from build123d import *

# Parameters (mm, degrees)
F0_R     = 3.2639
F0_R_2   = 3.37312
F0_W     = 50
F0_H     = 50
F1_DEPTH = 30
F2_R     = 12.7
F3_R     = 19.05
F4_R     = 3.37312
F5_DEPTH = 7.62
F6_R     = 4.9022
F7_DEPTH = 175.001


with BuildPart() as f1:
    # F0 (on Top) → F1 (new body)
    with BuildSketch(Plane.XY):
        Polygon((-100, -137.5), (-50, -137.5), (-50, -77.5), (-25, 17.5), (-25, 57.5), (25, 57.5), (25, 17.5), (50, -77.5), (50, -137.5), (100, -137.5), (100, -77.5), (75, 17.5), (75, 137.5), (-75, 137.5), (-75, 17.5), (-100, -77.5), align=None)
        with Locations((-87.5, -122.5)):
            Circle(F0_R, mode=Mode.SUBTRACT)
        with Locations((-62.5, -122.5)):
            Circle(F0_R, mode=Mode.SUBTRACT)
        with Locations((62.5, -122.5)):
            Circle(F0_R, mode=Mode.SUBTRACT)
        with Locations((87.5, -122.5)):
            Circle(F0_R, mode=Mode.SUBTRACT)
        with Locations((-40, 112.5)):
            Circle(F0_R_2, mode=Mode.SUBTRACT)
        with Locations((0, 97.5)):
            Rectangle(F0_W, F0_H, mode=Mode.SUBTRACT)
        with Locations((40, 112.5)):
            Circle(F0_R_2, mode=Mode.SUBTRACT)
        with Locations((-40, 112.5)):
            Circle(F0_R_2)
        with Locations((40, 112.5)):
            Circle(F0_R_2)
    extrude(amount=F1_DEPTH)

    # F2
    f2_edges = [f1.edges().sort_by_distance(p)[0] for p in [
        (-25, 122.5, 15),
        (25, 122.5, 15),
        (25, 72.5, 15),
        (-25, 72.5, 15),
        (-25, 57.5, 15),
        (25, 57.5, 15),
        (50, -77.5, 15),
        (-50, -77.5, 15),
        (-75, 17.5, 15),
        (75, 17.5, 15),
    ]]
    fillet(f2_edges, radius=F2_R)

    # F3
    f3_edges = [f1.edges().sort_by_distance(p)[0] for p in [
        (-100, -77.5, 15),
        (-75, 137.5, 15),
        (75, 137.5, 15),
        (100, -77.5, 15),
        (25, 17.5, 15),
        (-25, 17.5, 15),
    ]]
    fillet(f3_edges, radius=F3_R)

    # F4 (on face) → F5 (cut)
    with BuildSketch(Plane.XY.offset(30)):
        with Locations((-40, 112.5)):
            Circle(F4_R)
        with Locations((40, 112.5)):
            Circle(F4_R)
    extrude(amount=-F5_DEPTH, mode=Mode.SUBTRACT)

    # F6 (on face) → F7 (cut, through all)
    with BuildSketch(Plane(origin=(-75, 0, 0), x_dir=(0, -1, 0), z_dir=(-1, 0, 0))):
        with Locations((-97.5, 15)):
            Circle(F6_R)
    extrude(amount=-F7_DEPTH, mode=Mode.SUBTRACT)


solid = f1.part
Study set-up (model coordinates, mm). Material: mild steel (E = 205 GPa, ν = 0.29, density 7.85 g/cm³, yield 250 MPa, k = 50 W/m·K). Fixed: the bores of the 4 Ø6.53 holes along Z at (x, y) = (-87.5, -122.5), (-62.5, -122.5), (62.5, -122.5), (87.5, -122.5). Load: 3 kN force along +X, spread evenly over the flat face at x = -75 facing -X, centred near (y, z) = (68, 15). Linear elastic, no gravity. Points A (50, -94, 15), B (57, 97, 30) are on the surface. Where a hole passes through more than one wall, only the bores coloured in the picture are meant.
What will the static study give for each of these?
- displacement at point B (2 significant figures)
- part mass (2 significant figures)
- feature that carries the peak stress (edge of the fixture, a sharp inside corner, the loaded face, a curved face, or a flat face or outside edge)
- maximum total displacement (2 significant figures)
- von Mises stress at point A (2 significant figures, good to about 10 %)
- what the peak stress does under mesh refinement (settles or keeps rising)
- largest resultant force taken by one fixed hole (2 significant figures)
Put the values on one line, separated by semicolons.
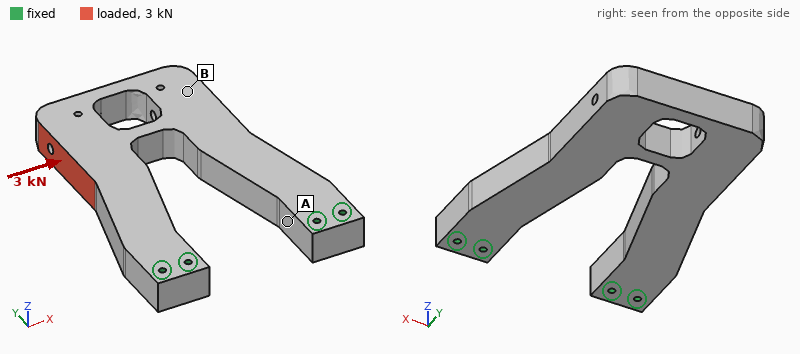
19 µm; 6.7 kg; edge of the fixture; 21 µm; 5.0 MPa; keeps rising; 5.7 kN
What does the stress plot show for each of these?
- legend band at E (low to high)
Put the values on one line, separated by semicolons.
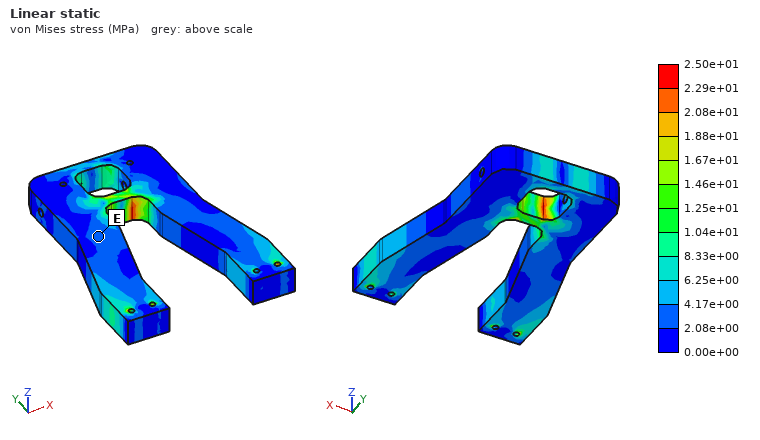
2.08e+00 to 4.17e+00 MPa
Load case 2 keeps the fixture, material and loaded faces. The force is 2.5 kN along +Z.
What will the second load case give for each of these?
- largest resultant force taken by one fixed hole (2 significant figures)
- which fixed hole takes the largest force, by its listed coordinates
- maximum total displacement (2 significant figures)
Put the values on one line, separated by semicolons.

1.6 kN; (-87.5, -122.5); 0.24 mm
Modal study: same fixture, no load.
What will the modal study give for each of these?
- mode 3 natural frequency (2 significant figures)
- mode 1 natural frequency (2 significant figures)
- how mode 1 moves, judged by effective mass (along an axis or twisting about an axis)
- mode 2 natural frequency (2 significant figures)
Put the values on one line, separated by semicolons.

1000 Hz; 330 Hz; along Z; 1000 Hz
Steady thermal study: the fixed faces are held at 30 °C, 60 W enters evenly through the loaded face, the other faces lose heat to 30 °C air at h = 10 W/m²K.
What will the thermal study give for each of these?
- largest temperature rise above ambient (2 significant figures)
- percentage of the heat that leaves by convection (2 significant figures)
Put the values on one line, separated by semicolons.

68 K; 45 %
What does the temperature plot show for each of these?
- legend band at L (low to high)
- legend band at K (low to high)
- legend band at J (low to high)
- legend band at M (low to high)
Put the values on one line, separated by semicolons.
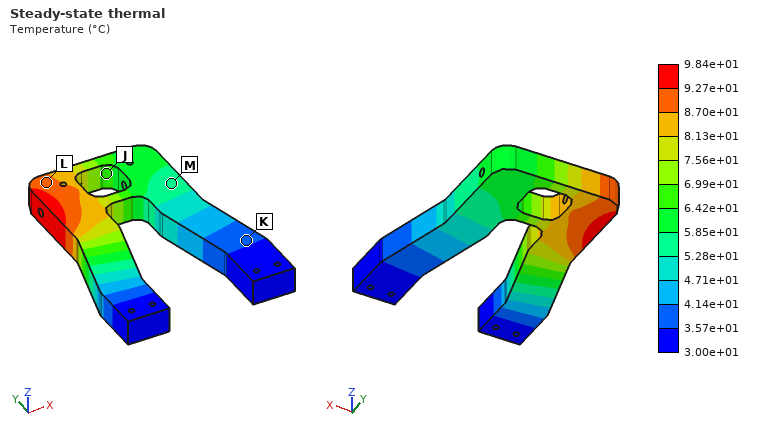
8.70e+01 to 9.27e+01 °C; 3.57e+01 to 4.14e+01 °C; 6.42e+01 to 6.99e+01 °C; 5.28e+01 to 5.85e+01 °C
